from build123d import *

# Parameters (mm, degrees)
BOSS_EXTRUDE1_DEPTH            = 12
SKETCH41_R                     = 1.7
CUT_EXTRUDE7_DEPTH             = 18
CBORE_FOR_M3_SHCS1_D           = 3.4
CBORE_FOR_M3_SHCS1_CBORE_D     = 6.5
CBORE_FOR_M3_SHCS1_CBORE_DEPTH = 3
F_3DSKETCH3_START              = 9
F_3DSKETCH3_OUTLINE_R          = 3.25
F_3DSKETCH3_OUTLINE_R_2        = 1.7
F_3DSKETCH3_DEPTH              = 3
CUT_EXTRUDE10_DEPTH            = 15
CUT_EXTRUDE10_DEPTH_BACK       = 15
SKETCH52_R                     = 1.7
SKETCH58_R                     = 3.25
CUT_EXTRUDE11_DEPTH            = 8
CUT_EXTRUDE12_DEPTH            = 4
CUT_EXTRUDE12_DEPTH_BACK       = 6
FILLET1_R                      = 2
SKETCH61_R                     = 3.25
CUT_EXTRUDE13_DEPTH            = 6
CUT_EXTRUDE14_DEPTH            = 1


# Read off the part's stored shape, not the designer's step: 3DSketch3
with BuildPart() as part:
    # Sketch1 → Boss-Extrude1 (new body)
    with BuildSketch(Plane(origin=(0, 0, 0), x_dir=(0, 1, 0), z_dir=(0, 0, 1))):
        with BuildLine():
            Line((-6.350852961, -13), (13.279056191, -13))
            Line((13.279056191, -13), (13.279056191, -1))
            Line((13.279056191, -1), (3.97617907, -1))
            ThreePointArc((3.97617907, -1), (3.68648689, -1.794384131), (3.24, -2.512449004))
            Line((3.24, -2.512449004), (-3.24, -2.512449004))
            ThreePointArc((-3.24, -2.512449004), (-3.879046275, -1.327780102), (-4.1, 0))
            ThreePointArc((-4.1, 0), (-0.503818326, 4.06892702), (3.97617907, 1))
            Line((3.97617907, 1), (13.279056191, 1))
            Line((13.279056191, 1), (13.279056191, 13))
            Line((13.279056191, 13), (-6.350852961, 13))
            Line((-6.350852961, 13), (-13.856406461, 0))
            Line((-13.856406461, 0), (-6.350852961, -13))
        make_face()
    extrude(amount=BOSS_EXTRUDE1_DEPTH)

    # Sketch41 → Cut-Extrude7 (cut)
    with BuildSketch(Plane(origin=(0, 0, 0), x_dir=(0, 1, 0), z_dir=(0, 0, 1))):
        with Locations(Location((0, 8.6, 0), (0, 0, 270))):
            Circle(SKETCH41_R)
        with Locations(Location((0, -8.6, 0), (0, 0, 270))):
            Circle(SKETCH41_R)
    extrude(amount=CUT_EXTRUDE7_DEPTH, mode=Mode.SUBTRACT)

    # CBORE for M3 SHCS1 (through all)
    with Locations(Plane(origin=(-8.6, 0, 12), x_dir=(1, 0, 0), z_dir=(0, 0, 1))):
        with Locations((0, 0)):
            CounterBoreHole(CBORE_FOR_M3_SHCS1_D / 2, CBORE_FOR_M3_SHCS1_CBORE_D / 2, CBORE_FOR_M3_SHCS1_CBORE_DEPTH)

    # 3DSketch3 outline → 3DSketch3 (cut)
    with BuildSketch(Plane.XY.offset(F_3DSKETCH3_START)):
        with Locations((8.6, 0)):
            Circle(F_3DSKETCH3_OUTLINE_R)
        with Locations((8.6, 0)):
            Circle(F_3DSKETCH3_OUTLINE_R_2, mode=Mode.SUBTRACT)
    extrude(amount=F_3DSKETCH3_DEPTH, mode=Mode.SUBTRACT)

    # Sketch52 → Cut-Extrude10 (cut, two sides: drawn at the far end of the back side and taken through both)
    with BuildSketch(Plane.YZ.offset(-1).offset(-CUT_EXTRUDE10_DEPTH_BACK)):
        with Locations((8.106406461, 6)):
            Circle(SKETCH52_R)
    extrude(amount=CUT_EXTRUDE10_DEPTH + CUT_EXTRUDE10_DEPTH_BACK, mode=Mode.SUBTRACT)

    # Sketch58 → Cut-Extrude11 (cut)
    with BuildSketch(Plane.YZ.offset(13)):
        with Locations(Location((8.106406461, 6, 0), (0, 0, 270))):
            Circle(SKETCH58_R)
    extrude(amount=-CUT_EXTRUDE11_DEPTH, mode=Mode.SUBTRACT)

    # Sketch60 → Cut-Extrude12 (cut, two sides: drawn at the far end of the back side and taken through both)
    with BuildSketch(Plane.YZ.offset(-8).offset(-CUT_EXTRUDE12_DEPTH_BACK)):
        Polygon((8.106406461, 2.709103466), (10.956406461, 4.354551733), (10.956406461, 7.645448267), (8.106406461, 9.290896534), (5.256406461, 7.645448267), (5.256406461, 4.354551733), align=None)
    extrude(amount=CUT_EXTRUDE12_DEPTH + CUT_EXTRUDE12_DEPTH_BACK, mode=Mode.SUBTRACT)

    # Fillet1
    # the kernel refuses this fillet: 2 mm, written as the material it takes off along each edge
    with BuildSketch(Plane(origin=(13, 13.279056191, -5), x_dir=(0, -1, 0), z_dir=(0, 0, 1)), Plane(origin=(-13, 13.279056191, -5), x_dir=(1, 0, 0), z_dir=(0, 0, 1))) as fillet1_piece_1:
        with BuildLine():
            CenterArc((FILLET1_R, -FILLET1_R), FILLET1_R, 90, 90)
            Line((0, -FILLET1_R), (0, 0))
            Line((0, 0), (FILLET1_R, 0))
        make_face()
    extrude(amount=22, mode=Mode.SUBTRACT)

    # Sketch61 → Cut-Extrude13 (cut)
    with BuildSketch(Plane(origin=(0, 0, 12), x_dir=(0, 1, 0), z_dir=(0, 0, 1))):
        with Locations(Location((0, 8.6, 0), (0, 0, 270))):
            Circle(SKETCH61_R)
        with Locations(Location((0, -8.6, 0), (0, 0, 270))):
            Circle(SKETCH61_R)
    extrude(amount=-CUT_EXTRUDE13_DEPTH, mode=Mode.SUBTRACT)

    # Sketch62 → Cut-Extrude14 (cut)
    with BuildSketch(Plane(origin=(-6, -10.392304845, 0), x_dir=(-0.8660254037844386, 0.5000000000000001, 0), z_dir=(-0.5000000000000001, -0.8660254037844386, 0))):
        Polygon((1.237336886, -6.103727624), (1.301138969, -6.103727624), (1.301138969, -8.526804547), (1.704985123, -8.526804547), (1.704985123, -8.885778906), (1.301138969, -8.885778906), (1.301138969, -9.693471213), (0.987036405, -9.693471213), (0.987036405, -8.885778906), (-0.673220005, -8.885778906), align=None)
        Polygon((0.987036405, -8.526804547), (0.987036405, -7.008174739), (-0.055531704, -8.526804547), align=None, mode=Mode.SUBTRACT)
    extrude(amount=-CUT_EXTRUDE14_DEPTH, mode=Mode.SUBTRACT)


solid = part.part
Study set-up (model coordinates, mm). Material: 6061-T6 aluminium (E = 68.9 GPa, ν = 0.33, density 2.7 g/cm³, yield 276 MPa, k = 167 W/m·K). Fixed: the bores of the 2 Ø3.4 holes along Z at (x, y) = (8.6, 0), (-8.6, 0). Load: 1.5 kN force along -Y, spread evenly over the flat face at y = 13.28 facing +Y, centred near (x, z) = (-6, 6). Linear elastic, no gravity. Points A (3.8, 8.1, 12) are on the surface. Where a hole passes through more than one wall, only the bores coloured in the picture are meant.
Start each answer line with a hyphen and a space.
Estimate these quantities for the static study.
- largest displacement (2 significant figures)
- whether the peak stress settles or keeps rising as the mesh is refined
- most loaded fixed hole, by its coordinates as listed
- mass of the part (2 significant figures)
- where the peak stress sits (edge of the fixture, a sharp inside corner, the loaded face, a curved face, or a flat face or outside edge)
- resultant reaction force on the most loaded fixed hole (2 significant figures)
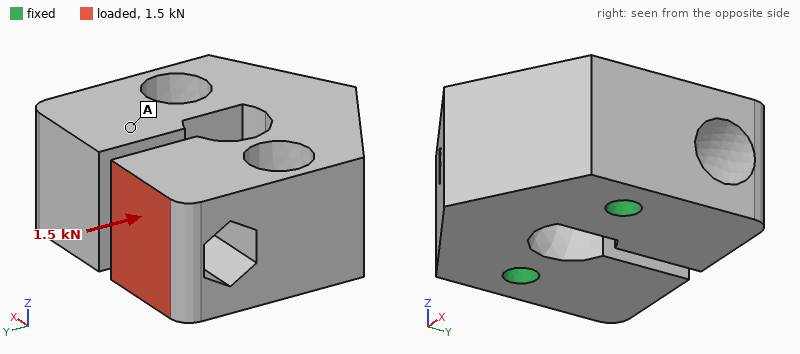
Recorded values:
- 19 µm
- keeps rising
- (-8.6, 0)
- 15 g
- edge of the fixture
- 1.4 kN
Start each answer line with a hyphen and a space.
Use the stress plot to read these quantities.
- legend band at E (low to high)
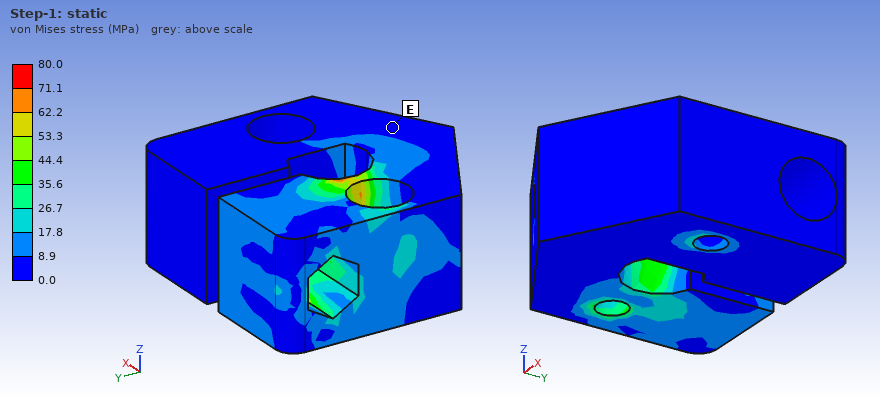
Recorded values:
- 0.0 to 8.9 MPa
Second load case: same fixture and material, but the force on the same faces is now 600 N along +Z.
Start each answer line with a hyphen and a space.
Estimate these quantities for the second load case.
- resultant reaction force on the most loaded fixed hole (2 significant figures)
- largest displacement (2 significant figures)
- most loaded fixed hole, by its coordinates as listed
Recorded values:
- 630 N
- 29 µm
- (-8.6, 0)
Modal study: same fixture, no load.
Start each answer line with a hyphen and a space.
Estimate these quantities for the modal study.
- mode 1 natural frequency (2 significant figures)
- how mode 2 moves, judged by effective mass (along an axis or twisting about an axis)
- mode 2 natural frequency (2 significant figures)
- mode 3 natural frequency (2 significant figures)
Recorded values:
- 17 kHz
- along X
- 19 kHz
- 21 kHz
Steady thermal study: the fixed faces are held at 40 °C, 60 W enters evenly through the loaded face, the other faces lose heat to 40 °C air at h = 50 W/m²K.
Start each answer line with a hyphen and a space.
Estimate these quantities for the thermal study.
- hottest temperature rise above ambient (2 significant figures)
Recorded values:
- 61 K
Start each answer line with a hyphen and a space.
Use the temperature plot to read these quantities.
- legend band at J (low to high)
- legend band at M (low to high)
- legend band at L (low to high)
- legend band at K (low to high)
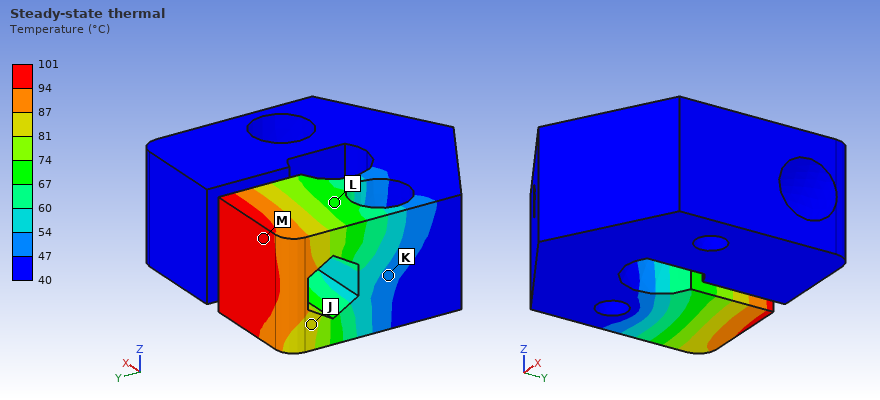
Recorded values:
- 81 to 87 °C
- 94 to 101 °C
- 67 to 74 °C
- 47 to 54 °C
